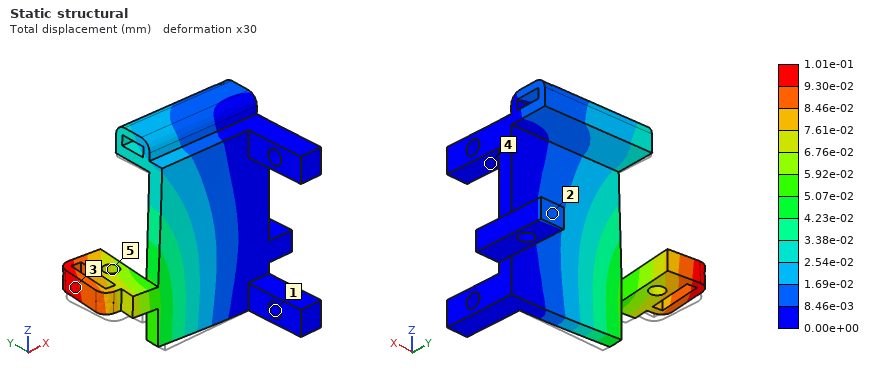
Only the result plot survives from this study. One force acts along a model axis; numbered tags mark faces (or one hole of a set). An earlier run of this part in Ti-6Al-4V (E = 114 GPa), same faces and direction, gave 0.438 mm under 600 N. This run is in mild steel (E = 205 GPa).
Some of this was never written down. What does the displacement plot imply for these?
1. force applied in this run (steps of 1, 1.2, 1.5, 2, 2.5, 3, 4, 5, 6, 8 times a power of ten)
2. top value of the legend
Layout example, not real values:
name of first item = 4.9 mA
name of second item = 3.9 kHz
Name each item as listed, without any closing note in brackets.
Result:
force applied in this run = 250 N
top value of the legend = 1.01e-01 mm
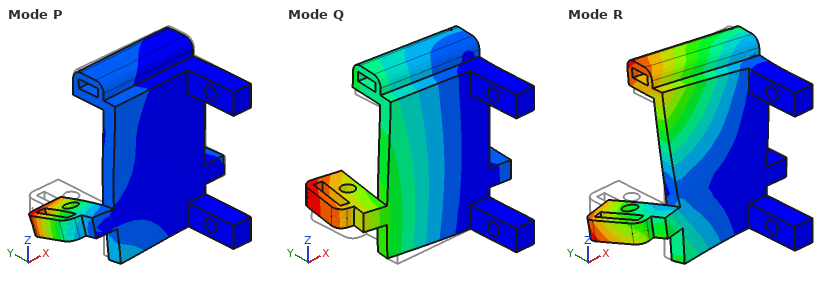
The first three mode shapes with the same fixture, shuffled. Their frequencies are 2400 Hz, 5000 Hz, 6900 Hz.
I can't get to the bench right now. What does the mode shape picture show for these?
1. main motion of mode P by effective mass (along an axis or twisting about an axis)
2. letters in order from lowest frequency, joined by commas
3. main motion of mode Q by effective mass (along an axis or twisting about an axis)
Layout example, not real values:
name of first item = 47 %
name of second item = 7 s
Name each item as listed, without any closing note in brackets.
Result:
main motion of mode P by effective mass = along Z
letters in order from lowest frequency, joined by commas = Q, R, P
main motion of mode Q by effective mass = along Y
